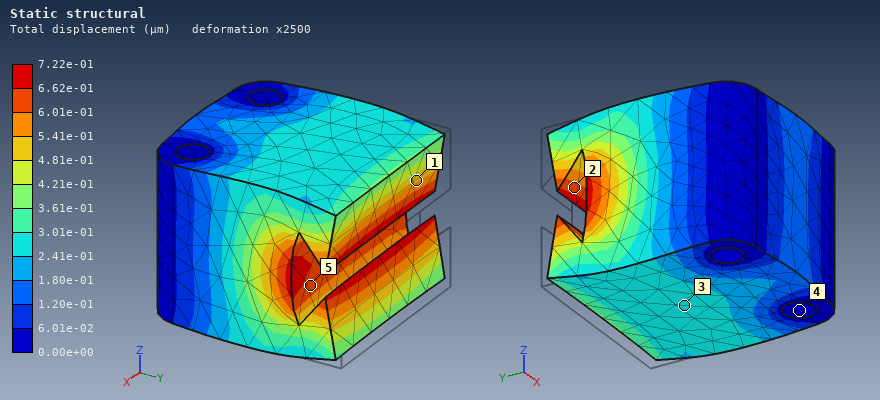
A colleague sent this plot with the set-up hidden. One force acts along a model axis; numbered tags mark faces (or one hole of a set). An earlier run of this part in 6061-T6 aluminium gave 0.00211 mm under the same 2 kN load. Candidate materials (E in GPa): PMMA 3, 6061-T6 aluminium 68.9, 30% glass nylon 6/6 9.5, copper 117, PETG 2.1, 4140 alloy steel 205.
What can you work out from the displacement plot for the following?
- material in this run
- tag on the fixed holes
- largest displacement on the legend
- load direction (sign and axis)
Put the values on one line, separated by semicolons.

4140 alloy steel; 4; 7.22e-01 µm; -Y
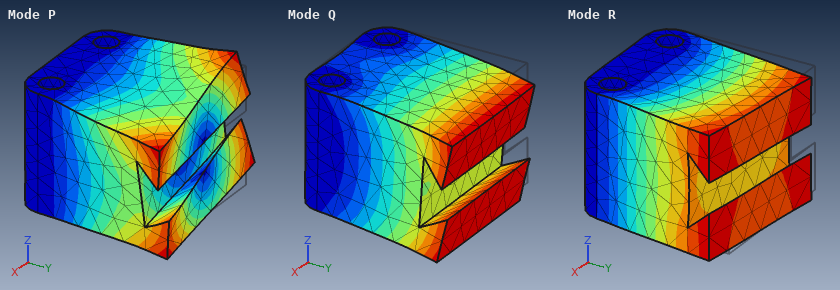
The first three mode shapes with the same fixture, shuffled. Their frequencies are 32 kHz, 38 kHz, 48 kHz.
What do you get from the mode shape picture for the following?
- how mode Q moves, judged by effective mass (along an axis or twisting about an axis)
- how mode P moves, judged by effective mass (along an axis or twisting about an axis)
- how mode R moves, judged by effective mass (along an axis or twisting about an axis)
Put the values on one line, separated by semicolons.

along Z; twisting about Y; along X
